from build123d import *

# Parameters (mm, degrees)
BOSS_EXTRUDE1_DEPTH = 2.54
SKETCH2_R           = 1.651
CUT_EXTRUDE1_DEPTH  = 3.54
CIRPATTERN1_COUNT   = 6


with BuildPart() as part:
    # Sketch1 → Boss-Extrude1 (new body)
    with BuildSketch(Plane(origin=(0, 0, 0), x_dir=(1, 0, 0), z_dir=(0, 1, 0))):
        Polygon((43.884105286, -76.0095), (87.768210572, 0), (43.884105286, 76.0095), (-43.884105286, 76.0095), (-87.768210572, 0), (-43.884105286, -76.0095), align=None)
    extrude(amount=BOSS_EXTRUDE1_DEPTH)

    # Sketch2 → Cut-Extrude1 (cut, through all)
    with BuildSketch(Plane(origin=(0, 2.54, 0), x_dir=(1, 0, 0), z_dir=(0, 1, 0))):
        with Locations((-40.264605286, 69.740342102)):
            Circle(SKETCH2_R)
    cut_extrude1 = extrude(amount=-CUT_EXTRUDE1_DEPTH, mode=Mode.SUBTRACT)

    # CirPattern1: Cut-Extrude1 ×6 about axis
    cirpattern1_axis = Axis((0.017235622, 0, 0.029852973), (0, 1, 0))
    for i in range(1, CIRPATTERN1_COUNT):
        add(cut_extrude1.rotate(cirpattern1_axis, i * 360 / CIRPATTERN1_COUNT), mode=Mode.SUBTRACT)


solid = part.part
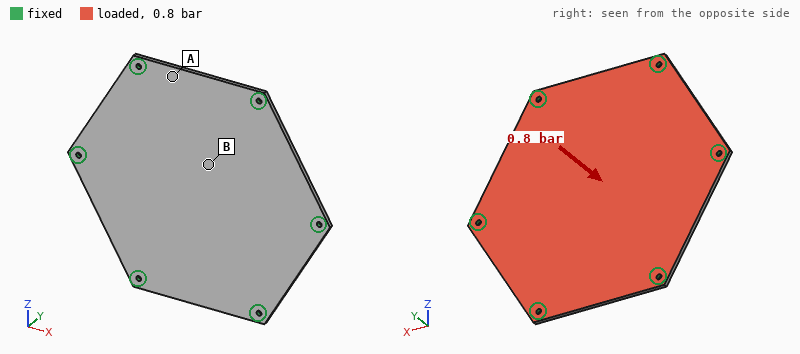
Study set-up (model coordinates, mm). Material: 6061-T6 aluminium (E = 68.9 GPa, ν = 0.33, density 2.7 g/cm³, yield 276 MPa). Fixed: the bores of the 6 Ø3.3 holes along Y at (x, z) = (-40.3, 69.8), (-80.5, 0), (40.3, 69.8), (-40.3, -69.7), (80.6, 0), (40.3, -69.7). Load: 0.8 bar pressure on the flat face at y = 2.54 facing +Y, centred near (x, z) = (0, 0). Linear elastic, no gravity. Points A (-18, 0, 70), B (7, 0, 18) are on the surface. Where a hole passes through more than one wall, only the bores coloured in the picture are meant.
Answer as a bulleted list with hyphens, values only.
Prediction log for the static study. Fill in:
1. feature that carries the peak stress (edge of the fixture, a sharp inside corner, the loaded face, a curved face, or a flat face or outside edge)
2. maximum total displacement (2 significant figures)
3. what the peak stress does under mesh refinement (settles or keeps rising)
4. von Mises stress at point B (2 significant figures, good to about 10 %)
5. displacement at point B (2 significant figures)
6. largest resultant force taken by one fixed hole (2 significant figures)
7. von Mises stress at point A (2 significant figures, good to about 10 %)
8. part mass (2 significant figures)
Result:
- edge of the fixture
- 0.87 mm
- keeps rising
- 50 MPa
- 0.79 mm
- 270 N
- 24 MPa
- 140 g
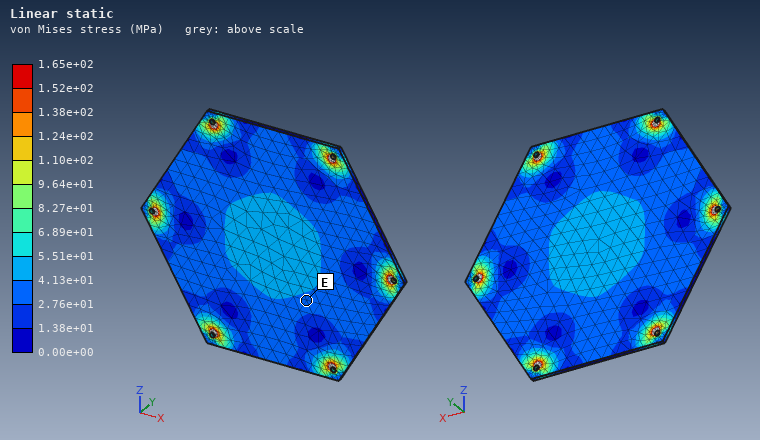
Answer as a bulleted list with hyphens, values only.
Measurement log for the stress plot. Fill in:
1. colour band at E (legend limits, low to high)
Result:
- 2.76e+01 to 4.13e+01 MPa
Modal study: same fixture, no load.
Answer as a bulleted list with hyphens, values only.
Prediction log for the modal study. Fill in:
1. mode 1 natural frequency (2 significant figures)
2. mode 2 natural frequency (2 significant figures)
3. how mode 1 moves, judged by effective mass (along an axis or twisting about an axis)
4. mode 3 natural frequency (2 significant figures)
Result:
- 730 Hz
- 1500 Hz
- along Y
- 1500 Hz
